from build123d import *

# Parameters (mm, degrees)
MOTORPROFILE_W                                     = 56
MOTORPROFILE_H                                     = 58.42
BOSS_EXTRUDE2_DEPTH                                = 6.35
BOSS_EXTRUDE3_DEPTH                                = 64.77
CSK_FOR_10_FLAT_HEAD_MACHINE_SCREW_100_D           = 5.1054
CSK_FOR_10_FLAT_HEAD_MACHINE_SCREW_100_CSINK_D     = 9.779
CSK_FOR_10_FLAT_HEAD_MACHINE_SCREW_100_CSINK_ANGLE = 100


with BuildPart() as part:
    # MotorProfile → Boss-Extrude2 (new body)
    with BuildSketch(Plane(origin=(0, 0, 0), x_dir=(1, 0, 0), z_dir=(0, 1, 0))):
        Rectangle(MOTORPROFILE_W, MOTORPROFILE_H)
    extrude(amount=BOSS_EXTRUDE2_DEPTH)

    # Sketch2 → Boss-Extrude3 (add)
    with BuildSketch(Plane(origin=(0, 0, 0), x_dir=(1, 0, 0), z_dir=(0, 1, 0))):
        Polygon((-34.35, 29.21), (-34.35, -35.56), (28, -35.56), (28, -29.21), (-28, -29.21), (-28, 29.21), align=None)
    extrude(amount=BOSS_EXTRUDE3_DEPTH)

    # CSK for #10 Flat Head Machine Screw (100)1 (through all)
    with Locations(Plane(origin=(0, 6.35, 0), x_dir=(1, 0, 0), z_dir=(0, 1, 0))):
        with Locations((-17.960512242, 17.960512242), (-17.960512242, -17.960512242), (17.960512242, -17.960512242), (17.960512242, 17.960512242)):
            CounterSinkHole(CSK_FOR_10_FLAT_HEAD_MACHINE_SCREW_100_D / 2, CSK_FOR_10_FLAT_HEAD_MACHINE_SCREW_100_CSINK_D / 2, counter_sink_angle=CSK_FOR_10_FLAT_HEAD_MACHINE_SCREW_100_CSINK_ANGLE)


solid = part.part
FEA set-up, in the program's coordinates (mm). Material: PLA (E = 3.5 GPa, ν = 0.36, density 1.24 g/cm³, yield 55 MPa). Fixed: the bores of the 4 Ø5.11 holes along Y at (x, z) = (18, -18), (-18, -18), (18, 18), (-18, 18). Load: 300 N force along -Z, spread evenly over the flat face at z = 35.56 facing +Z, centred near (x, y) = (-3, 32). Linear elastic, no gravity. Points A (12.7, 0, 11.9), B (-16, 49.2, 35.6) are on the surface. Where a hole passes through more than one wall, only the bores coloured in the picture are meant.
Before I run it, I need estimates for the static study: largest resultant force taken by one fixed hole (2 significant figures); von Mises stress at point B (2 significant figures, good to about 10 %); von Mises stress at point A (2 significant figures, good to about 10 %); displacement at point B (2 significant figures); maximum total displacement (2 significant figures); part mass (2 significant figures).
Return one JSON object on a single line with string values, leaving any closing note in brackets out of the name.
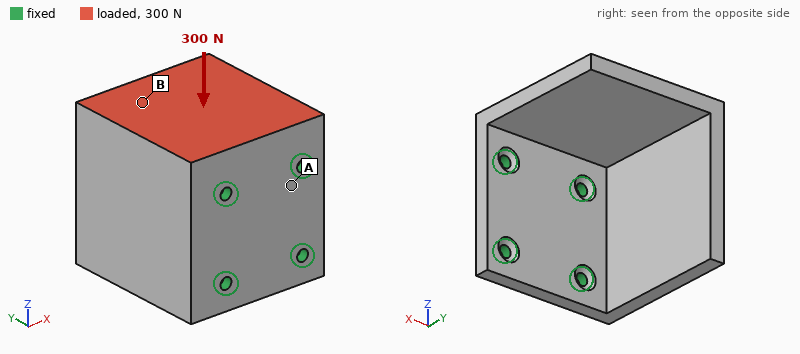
{"largest resultant force taken by one fixed hole": "230 N", "von Mises stress at point B": "4.3 MPa", "von Mises stress at point A": "1.3 MPa", "displacement at point B": "0.38 mm", "maximum total displacement": "1.2 mm", "part mass": "86 g"}
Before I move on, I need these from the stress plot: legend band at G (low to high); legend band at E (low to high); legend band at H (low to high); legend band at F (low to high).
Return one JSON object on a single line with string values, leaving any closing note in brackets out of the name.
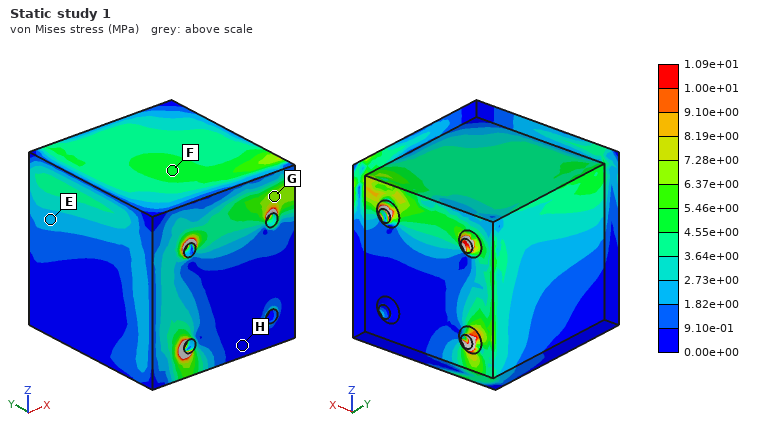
{"legend band at G": "6.37e+00 to 7.28e+00 MPa", "legend band at E": "1.82e+00 to 2.73e+00 MPa", "legend band at H": "0.00e+00 to 9.10e-01 MPa", "legend band at F": "4.55e+00 to 5.46e+00 MPa"}
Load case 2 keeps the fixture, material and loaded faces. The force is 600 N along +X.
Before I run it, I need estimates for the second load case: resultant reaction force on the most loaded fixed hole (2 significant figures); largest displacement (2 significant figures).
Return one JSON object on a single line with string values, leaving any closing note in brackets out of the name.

{"resultant reaction force on the most loaded fixed hole": "610 N", "largest displacement": "0.58 mm"}
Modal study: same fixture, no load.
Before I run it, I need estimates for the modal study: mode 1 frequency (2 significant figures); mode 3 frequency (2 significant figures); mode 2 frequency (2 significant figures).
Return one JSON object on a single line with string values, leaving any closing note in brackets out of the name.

{"mode 1 frequency": "520 Hz", "mode 3 frequency": "980 Hz", "mode 2 frequency": "700 Hz"}
